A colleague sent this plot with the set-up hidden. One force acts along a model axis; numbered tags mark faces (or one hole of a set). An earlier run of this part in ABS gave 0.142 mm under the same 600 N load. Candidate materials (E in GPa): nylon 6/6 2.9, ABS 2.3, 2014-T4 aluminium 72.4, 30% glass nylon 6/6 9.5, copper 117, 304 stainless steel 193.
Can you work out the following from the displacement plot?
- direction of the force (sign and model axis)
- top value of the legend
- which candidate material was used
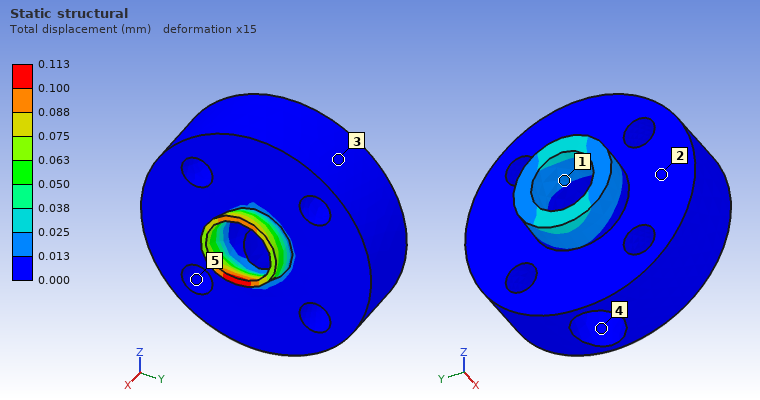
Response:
+Z
0.113 mm
nylon 6/6
